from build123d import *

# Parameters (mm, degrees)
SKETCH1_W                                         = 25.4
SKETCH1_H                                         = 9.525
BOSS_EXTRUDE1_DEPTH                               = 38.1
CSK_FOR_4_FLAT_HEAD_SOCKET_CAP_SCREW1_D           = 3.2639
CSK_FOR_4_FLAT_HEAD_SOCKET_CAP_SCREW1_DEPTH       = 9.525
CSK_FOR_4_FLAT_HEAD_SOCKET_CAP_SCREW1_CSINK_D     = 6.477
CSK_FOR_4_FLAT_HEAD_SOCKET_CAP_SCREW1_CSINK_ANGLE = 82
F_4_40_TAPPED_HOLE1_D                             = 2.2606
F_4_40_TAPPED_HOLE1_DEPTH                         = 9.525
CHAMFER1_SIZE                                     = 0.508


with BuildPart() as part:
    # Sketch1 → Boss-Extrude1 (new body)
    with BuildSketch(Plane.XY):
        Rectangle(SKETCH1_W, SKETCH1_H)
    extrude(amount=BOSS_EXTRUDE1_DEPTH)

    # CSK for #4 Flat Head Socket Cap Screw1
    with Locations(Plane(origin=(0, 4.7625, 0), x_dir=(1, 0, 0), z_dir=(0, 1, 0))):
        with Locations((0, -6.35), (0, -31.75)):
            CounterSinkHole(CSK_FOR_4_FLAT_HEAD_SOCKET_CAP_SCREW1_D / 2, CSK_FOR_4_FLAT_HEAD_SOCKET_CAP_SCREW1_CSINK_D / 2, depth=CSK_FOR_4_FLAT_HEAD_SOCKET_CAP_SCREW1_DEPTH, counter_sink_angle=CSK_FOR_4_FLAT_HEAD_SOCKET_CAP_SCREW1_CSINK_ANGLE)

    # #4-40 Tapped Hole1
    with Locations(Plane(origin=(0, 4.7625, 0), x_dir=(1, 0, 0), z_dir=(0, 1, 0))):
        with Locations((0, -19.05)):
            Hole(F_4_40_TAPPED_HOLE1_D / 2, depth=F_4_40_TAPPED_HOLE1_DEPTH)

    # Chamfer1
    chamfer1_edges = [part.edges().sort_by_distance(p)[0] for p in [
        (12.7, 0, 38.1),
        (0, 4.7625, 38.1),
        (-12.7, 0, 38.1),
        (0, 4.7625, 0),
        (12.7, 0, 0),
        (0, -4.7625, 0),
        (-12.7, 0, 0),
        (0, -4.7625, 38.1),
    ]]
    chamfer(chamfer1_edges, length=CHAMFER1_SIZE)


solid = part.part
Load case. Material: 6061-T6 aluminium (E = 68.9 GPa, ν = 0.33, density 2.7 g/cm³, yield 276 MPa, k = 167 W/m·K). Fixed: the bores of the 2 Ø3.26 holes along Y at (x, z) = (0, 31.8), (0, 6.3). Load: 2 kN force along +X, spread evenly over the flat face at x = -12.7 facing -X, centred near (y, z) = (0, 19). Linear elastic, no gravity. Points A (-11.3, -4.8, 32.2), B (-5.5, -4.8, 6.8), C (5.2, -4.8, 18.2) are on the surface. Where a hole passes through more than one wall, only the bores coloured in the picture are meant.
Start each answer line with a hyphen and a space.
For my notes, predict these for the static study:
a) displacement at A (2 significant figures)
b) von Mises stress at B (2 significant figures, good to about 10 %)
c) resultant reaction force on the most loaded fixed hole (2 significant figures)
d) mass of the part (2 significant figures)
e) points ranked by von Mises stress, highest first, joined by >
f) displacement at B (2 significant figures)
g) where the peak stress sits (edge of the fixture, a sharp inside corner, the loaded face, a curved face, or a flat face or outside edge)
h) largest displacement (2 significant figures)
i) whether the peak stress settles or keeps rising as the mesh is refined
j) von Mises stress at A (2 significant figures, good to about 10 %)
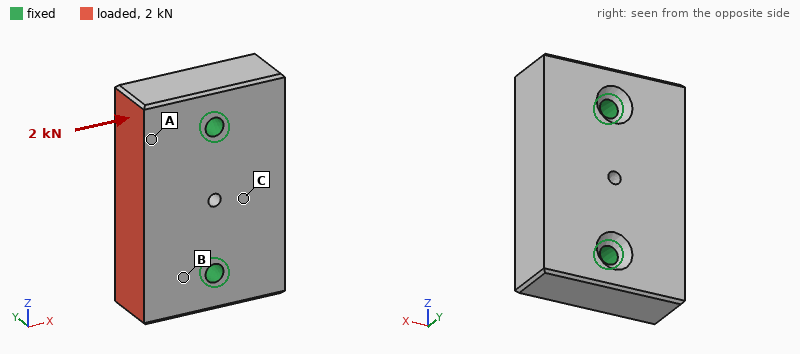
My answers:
- 1.1 µm
- 8.1 MPa
- 1.0 kN
- 24 g
- B > A > C
- 0.50 µm
- edge of the fixture
- 2.4 µm
- keeps rising
- 5.8 MPa
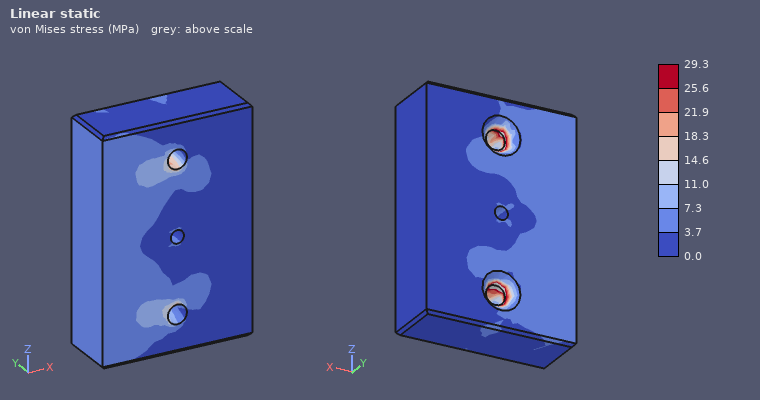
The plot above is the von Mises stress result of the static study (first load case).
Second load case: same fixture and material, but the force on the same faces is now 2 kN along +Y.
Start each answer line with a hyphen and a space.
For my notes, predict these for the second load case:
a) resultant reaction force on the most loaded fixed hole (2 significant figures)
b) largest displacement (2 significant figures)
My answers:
- 1.0 kN
- 24 µm
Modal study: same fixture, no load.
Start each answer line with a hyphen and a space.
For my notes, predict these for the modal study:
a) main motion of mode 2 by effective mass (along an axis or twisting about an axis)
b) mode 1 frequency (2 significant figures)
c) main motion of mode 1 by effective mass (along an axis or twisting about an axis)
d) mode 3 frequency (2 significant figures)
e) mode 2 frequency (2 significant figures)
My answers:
- along Y
- 21 kHz
- twisting about Z
- 34 kHz
- 28 kHz
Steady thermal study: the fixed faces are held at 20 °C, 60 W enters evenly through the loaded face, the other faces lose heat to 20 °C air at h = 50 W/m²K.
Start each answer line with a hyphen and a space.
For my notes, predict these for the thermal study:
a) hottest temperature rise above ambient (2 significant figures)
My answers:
- 16 K
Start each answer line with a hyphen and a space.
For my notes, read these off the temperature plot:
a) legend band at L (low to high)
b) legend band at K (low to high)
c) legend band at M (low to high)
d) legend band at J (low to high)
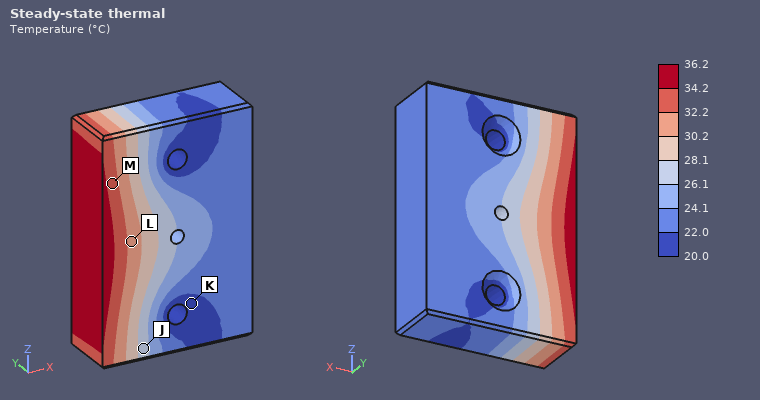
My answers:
- 30.2 to 32.2 °C
- 20.0 to 22.0 °C
- 32.2 to 34.2 °C
- 26.1 to 28.1 °C
